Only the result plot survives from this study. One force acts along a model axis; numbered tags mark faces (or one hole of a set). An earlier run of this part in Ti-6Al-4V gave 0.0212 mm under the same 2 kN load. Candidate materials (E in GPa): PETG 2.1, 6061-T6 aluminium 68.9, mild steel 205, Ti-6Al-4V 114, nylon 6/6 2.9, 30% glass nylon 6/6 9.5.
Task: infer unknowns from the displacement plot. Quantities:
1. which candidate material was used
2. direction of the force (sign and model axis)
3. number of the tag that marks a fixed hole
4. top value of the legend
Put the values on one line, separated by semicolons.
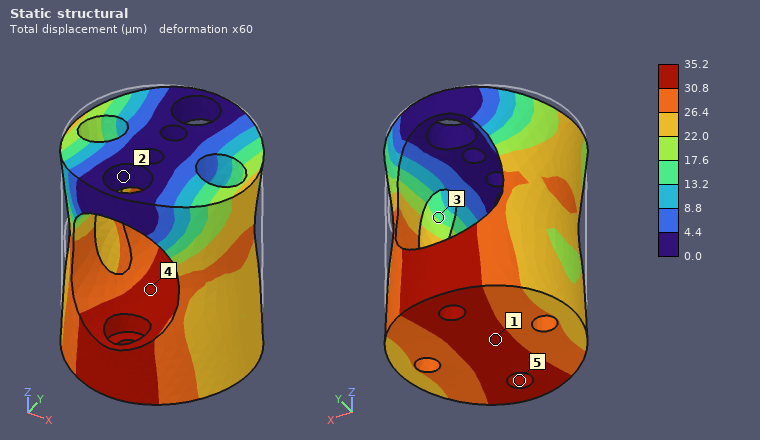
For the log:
6061-T6 aluminium; -Z; 2; 35.2 µm
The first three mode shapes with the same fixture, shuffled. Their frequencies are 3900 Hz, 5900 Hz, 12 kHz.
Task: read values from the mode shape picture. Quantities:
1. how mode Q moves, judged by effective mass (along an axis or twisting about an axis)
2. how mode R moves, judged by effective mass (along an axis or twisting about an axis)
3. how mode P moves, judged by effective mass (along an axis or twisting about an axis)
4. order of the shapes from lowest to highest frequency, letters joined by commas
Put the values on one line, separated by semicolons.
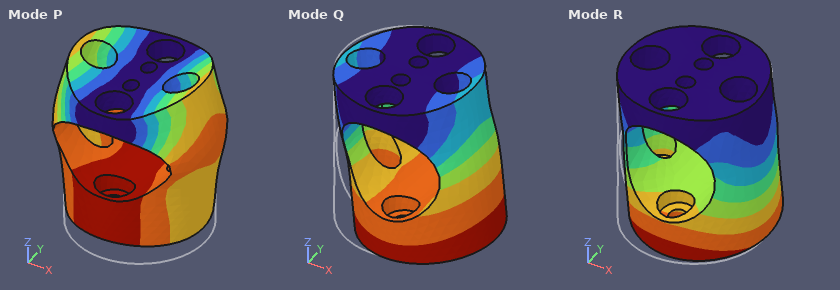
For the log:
along X; along Y; along Z; Q, R, P
